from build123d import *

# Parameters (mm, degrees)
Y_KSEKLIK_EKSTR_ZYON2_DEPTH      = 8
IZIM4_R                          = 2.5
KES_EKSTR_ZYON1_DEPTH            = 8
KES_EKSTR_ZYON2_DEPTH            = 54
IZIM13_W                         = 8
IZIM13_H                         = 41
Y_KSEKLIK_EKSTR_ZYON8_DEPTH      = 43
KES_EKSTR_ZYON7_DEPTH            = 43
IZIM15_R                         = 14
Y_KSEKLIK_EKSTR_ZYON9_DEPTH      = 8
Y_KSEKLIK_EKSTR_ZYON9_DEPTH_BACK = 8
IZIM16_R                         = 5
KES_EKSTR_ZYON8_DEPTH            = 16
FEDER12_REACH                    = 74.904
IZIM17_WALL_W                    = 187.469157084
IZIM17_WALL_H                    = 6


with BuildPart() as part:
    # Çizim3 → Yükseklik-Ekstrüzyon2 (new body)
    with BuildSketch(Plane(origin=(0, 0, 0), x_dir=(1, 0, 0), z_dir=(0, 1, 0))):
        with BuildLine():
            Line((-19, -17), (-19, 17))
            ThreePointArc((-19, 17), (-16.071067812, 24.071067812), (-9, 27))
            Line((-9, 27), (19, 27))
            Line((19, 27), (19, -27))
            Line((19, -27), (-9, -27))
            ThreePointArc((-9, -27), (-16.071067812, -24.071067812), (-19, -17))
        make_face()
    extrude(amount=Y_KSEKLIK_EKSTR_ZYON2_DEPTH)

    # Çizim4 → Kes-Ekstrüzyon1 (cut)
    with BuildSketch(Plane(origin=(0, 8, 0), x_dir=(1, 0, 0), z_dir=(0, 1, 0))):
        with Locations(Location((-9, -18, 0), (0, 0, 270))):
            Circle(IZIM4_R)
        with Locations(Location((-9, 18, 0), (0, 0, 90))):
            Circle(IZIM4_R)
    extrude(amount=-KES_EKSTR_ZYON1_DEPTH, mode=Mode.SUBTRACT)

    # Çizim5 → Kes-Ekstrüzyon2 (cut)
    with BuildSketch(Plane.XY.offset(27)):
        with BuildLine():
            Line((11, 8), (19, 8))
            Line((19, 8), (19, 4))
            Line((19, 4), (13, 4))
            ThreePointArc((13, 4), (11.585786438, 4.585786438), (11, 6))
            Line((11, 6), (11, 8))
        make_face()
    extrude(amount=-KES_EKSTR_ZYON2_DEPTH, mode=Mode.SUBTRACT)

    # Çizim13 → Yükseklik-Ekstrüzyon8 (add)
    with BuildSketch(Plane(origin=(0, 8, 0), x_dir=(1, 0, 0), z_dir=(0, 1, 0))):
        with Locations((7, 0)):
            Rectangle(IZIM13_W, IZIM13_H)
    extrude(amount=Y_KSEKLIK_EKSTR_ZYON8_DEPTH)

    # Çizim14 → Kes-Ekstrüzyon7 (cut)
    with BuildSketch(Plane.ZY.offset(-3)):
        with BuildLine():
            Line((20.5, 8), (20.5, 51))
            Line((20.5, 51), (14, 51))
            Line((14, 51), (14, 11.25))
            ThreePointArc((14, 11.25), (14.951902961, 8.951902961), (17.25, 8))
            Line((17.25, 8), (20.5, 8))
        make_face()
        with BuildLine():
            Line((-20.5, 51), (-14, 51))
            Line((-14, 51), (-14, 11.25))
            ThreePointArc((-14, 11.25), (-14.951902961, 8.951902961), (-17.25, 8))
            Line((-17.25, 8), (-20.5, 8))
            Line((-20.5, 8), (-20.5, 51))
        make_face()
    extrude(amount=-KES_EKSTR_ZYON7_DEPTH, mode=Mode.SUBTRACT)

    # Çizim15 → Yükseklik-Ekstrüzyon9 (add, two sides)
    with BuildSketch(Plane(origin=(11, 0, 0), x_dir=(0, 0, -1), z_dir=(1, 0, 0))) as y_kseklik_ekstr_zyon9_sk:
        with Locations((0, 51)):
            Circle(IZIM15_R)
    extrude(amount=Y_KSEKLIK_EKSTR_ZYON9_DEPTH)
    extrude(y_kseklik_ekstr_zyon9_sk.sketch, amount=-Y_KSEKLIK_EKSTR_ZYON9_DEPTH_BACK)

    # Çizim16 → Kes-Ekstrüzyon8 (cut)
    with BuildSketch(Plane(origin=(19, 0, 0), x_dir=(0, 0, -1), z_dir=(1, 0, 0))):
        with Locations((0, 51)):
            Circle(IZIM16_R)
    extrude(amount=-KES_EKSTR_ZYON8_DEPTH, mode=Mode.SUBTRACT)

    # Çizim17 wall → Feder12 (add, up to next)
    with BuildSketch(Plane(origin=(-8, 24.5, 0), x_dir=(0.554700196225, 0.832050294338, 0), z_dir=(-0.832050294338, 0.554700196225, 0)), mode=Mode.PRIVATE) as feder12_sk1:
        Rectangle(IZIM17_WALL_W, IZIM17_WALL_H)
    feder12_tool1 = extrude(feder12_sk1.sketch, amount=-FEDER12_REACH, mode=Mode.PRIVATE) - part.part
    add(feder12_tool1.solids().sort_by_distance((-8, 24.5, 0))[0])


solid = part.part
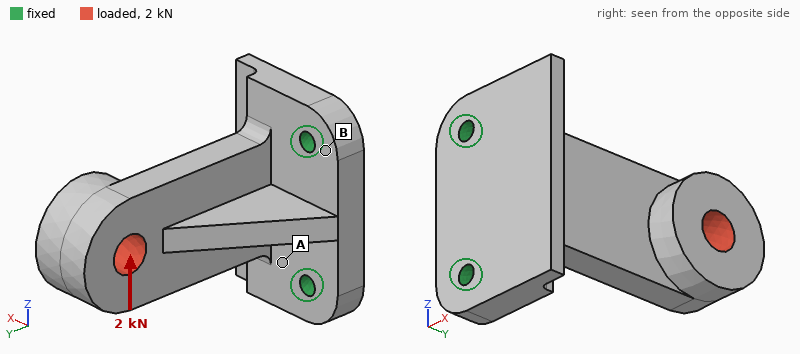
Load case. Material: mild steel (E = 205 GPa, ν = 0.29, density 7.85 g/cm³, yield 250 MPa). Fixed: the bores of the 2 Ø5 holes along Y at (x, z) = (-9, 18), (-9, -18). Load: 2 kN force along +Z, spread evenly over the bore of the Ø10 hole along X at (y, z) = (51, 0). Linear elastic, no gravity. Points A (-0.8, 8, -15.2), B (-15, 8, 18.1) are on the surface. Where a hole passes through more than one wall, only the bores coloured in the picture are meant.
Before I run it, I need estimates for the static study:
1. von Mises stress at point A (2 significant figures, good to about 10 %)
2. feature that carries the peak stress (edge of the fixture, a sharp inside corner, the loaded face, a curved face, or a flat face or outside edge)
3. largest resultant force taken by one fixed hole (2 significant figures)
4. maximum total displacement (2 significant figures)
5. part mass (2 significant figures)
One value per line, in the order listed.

41 MPa
a curved face
3.1 kN
84 µm
250 g
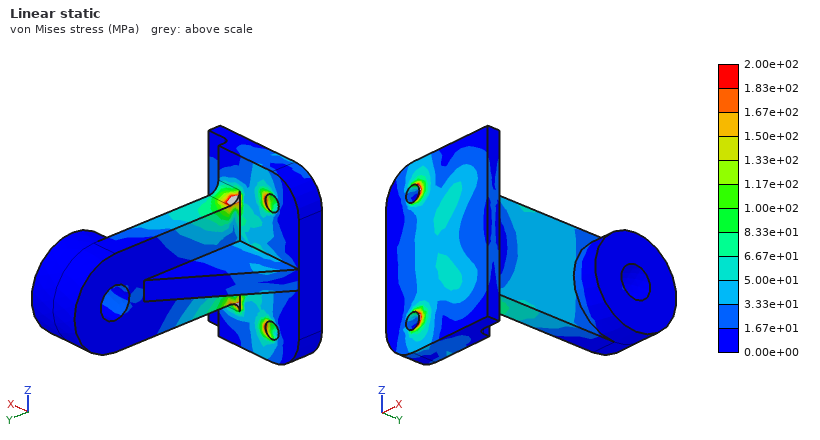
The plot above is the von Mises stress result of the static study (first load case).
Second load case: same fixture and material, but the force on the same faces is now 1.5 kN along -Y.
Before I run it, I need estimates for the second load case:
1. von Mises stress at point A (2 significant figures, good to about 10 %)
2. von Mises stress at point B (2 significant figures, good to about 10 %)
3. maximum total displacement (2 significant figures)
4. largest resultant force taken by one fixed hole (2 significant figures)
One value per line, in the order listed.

25 MPa
13 MPa
49 µm
760 N
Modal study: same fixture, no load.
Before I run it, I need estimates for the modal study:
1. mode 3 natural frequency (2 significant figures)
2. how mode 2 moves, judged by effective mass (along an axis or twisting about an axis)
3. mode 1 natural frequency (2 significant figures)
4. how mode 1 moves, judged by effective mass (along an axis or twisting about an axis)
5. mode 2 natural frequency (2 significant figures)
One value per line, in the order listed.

6900 Hz
along Z
2000 Hz
along X
3100 Hz
